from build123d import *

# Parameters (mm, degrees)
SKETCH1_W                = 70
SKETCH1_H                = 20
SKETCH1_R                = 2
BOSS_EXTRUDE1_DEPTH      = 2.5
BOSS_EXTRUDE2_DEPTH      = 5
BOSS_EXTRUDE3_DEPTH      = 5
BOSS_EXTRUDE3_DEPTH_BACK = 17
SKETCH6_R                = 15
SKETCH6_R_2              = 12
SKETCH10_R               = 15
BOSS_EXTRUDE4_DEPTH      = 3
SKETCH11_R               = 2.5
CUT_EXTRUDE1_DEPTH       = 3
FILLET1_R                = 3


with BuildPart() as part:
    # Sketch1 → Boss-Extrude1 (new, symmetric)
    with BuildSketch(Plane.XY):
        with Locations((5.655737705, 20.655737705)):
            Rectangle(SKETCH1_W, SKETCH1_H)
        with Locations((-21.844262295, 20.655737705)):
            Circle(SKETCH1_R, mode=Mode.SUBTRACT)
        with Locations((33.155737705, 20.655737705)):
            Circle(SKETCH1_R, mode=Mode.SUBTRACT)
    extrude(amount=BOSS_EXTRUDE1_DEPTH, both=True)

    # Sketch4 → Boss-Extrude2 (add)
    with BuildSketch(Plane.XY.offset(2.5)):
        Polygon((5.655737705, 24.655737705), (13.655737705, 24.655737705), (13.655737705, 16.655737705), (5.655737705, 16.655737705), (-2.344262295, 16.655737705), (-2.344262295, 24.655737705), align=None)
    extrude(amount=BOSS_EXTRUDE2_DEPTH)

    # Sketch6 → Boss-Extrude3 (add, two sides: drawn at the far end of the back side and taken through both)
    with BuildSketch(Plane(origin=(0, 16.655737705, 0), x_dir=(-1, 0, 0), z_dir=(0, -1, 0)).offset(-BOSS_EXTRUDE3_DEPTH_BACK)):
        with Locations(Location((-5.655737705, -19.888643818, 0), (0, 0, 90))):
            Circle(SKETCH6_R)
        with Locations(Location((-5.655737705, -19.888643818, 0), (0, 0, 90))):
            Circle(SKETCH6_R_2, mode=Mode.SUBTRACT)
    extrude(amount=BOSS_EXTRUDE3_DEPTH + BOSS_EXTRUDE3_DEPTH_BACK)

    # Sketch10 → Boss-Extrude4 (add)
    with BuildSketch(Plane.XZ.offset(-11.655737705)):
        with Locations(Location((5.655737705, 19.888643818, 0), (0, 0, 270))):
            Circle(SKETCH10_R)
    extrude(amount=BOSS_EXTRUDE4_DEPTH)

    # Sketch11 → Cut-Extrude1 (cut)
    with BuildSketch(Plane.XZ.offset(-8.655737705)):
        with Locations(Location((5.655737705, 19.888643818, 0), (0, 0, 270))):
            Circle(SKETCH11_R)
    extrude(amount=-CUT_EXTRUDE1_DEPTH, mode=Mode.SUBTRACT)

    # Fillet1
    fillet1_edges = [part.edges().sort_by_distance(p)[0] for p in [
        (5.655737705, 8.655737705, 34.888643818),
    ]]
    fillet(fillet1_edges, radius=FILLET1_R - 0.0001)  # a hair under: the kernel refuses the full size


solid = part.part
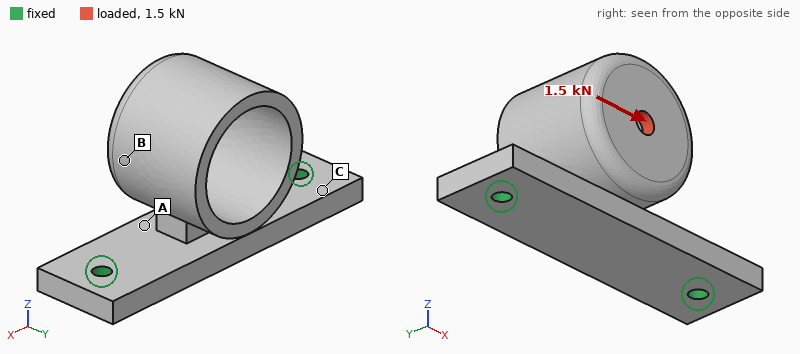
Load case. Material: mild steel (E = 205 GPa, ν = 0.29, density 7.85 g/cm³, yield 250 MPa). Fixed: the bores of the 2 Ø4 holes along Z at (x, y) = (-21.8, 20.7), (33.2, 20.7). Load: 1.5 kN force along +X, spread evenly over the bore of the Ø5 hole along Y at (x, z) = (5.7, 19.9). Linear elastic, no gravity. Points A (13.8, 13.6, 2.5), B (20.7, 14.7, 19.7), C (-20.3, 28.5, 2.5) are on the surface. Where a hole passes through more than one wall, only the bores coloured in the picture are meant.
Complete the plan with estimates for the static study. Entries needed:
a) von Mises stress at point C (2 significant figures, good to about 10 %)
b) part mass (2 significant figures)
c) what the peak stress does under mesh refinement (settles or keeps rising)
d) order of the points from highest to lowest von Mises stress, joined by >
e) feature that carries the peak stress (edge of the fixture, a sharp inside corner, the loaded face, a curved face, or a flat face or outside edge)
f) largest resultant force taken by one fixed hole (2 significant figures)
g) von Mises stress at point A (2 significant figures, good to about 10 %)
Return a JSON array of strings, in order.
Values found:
["23 MPa", "120 g", "keeps rising", "A > C > B", "edge of the fixture", "1.1 kN", "87 MPa"]
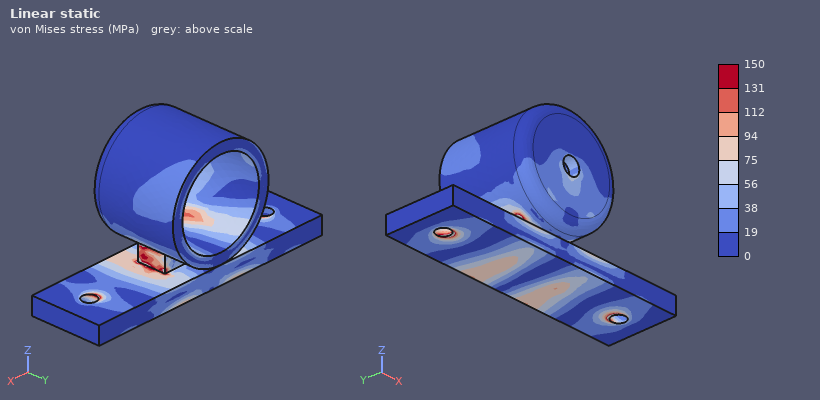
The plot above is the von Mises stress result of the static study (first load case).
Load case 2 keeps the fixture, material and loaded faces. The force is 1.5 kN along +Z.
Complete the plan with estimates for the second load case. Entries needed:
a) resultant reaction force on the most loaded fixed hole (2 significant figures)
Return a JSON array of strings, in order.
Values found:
["780 N"]
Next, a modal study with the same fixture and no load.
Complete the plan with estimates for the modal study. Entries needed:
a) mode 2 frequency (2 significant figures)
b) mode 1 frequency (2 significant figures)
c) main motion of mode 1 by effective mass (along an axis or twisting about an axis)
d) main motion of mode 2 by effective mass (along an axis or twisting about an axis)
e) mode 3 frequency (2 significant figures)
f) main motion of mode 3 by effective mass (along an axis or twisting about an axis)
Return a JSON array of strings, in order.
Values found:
["2900 Hz", "1800 Hz", "along Y", "along X", "4400 Hz", "along Z"]
